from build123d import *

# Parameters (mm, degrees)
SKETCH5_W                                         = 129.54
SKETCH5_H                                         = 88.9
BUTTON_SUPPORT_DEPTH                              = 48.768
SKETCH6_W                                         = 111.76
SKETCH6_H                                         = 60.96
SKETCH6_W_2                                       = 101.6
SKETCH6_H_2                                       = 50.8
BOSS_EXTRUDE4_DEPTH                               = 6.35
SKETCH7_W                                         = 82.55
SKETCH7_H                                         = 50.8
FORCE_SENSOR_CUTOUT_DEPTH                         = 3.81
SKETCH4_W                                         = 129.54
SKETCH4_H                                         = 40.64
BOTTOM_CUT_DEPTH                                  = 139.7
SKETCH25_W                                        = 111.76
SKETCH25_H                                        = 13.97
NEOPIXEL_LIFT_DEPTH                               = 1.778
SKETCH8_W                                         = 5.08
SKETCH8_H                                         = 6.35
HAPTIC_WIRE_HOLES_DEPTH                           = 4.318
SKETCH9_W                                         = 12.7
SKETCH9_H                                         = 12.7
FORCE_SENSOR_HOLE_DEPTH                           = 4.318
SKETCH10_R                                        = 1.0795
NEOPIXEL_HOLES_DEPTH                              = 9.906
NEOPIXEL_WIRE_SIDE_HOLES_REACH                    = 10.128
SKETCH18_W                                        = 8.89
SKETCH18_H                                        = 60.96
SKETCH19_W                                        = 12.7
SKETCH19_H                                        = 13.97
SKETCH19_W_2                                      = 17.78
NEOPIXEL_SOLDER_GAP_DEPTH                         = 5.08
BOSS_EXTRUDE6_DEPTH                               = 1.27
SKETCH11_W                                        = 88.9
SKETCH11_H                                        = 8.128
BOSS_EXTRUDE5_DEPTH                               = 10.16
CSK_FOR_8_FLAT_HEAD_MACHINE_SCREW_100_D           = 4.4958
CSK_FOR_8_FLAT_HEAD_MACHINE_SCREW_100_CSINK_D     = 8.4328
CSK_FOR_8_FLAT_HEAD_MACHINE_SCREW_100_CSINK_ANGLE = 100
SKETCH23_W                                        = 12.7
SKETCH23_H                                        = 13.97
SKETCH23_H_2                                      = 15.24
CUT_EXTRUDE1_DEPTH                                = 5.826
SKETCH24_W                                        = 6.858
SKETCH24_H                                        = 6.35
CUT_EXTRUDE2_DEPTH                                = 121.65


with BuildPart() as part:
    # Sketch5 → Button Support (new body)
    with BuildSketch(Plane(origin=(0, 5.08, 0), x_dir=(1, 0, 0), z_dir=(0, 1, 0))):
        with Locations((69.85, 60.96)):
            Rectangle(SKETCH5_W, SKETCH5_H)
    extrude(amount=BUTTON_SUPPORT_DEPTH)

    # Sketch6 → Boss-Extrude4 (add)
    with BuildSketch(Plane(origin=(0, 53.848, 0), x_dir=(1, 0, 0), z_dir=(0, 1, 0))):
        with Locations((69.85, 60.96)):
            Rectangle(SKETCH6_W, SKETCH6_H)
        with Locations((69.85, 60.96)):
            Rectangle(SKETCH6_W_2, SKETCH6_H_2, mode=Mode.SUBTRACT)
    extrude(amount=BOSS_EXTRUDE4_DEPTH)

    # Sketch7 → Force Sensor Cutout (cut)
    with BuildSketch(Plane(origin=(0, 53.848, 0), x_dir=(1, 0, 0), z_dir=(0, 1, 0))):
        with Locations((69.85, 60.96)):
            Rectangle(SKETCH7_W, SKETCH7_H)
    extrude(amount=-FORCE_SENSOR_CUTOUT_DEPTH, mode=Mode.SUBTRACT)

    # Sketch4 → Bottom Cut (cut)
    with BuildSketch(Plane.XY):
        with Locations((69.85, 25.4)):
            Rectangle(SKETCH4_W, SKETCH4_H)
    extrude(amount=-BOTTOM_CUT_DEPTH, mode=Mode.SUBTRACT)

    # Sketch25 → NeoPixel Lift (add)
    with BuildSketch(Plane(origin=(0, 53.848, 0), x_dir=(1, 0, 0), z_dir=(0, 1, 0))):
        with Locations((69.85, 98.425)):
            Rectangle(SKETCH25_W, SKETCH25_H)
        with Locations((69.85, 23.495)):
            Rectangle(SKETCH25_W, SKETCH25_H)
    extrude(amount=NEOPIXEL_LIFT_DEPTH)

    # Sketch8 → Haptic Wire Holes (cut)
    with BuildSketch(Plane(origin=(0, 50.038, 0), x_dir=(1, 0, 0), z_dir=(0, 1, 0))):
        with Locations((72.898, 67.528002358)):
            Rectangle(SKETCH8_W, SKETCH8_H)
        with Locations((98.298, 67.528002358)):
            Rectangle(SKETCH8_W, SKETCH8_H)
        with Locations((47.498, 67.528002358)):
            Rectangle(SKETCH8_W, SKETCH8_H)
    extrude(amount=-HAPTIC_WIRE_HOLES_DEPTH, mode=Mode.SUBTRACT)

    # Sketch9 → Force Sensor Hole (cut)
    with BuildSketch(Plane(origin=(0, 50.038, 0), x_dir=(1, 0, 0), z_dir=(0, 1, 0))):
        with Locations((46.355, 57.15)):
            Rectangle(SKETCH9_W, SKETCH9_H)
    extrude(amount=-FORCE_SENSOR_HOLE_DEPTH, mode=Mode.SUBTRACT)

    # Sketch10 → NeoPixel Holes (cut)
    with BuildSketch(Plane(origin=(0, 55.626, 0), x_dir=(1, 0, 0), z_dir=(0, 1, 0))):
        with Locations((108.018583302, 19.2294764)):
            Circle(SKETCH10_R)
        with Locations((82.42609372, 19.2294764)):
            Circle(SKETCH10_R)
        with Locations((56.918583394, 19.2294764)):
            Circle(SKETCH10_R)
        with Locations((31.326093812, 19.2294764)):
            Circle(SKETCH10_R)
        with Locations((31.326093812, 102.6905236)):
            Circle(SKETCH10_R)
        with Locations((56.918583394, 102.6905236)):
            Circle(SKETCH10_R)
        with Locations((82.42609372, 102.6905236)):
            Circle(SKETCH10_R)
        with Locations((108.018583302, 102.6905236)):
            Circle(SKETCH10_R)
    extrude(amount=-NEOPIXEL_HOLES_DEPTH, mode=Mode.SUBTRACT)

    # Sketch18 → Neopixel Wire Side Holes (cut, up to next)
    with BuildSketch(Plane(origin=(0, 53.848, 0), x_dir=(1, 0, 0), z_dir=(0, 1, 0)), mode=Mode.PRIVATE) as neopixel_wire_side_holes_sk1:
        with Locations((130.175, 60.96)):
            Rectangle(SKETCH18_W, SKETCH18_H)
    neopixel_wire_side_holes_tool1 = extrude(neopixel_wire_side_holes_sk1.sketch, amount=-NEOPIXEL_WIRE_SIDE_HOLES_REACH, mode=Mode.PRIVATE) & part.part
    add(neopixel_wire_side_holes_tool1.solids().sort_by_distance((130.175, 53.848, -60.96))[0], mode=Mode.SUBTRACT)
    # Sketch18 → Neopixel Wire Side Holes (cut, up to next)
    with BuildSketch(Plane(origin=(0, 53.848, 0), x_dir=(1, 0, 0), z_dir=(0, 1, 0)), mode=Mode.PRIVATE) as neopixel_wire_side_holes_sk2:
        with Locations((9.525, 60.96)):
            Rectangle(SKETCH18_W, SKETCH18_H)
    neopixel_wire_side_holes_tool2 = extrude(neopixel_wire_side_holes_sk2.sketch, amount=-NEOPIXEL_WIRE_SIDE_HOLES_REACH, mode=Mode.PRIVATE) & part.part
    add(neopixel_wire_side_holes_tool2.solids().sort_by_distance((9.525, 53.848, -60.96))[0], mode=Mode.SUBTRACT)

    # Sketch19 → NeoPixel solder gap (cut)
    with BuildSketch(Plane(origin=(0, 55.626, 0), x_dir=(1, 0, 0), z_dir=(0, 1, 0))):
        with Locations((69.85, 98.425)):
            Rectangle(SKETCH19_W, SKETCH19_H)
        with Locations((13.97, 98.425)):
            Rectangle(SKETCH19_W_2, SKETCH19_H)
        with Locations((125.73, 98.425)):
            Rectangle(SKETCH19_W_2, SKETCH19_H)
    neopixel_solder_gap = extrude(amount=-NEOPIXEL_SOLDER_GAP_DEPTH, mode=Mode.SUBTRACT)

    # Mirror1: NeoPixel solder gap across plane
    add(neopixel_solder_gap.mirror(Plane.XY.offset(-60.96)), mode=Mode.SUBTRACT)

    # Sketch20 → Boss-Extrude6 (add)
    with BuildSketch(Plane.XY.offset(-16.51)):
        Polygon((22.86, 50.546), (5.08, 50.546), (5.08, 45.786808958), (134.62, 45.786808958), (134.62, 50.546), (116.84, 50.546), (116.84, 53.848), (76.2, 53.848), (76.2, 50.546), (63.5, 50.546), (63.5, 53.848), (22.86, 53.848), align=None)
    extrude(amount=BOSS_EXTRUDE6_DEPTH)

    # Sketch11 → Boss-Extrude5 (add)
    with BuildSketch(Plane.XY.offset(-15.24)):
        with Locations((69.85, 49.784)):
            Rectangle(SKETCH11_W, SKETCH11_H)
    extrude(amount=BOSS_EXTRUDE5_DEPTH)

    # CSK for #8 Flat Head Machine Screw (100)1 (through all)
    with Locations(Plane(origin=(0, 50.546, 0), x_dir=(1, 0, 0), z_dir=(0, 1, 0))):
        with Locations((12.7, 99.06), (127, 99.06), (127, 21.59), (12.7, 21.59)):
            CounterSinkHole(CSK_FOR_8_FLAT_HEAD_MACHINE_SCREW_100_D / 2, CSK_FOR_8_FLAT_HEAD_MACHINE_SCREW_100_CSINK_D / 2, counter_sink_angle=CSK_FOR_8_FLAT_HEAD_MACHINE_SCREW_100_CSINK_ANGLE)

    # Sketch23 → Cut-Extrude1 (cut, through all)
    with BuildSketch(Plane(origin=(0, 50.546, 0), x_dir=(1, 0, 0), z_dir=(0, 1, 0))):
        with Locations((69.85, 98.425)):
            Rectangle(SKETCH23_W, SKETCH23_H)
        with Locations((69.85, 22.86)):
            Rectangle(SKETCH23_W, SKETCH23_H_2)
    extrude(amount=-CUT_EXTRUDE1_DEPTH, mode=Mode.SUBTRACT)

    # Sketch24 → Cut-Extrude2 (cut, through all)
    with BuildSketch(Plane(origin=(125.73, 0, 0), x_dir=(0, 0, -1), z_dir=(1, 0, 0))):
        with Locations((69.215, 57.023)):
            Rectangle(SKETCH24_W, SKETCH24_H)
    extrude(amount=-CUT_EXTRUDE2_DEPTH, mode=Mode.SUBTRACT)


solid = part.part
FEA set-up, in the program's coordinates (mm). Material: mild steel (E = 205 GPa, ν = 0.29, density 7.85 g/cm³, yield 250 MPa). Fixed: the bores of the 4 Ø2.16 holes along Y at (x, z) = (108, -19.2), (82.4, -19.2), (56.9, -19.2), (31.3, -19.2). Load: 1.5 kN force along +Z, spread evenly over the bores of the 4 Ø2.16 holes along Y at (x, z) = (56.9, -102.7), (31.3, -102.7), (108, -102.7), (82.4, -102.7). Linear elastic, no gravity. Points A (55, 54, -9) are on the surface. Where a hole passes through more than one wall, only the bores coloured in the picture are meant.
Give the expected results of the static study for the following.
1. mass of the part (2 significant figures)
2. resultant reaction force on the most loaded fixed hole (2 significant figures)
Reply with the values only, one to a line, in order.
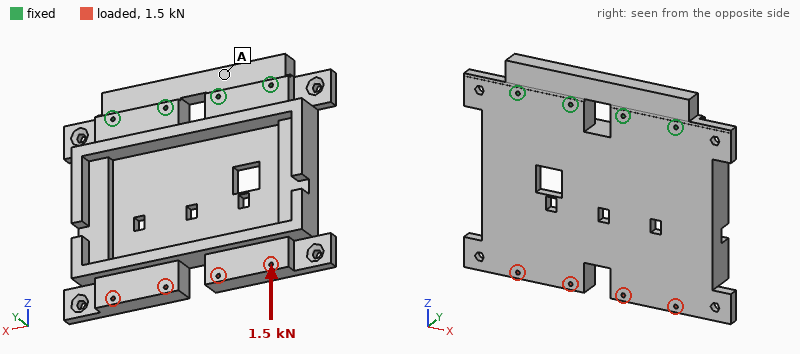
650 g
530 N
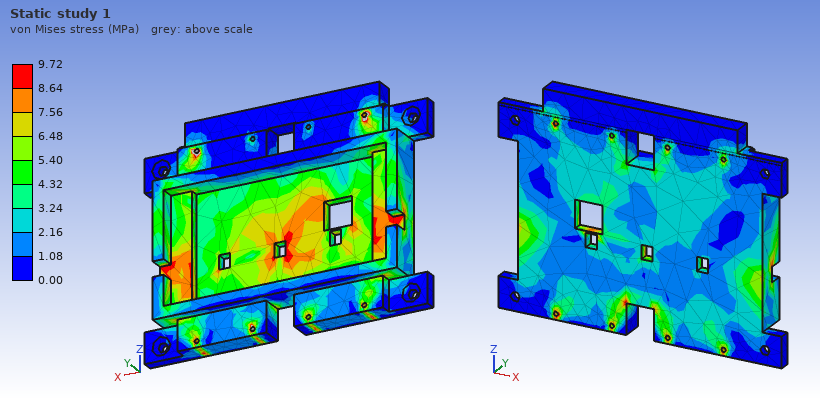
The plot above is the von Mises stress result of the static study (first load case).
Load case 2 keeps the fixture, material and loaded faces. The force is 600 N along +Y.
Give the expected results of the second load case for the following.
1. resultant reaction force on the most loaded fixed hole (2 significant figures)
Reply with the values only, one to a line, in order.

570 N
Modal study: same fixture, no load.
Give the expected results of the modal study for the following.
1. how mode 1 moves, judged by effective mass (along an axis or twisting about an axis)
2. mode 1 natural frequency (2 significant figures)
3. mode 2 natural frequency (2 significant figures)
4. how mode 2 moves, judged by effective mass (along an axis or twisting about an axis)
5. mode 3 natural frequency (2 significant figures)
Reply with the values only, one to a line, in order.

along Y
720 Hz
1300 Hz
twisting about Z
4100 Hz
